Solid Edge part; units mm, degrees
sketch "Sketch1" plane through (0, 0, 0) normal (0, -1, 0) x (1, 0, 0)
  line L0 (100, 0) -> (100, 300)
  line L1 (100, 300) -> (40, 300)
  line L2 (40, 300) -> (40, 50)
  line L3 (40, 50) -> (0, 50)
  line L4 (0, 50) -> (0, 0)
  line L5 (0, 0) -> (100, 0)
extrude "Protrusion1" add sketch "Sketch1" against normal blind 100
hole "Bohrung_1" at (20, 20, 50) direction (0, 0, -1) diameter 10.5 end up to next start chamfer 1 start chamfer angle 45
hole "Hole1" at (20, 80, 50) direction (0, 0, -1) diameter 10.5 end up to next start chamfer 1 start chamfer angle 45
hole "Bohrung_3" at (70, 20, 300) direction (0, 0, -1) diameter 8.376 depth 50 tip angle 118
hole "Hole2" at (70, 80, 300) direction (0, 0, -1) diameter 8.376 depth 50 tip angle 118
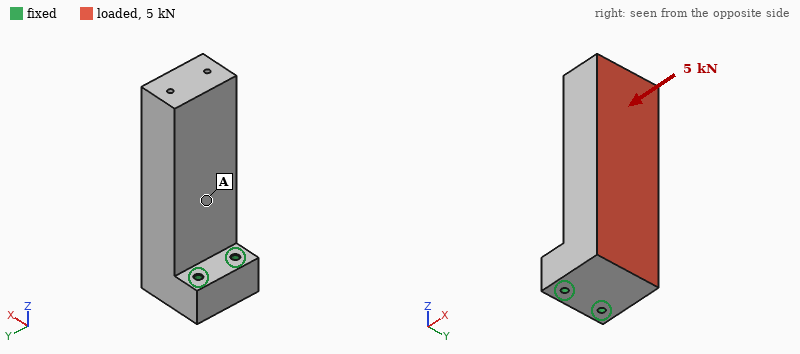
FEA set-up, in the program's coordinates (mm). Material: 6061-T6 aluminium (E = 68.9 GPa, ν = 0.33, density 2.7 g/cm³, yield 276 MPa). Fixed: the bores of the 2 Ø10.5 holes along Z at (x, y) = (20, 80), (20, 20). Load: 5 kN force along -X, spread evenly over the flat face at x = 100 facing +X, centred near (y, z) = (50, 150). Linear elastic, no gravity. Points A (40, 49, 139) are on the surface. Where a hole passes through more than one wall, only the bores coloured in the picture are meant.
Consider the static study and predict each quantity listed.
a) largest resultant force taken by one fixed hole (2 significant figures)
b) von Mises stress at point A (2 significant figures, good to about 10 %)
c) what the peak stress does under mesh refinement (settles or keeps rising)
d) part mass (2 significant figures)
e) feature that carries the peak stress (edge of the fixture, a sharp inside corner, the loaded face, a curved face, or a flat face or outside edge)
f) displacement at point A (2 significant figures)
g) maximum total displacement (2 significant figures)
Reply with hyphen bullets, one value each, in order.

- 2.6 kN
- 3.6 MPa
- keeps rising
- 5.4 kg
- edge of the fixture
- 0.067 mm
- 0.20 mm
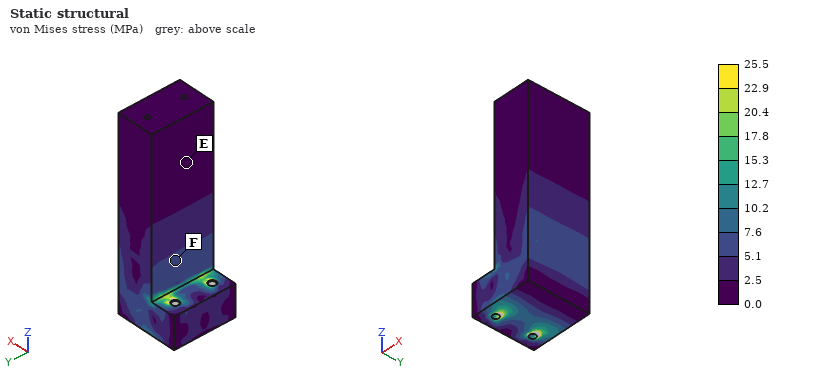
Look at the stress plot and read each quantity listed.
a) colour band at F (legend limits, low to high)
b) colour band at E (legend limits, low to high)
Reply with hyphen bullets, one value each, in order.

- 5.1 to 7.6 MPa
- 0.0 to 2.5 MPa
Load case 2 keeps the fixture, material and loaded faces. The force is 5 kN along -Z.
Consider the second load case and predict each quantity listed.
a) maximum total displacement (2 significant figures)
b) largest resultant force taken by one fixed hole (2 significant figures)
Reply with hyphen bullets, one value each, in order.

- 90 µm
- 2.5 kN
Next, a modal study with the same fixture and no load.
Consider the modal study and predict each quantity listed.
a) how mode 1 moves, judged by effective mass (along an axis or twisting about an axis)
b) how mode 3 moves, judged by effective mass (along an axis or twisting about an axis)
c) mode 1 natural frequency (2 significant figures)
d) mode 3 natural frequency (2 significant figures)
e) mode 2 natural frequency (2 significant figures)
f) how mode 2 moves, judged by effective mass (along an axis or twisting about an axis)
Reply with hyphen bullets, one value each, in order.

- along X
- twisting about Z
- 440 Hz
- 2200 Hz
- 660 Hz
- along Y
